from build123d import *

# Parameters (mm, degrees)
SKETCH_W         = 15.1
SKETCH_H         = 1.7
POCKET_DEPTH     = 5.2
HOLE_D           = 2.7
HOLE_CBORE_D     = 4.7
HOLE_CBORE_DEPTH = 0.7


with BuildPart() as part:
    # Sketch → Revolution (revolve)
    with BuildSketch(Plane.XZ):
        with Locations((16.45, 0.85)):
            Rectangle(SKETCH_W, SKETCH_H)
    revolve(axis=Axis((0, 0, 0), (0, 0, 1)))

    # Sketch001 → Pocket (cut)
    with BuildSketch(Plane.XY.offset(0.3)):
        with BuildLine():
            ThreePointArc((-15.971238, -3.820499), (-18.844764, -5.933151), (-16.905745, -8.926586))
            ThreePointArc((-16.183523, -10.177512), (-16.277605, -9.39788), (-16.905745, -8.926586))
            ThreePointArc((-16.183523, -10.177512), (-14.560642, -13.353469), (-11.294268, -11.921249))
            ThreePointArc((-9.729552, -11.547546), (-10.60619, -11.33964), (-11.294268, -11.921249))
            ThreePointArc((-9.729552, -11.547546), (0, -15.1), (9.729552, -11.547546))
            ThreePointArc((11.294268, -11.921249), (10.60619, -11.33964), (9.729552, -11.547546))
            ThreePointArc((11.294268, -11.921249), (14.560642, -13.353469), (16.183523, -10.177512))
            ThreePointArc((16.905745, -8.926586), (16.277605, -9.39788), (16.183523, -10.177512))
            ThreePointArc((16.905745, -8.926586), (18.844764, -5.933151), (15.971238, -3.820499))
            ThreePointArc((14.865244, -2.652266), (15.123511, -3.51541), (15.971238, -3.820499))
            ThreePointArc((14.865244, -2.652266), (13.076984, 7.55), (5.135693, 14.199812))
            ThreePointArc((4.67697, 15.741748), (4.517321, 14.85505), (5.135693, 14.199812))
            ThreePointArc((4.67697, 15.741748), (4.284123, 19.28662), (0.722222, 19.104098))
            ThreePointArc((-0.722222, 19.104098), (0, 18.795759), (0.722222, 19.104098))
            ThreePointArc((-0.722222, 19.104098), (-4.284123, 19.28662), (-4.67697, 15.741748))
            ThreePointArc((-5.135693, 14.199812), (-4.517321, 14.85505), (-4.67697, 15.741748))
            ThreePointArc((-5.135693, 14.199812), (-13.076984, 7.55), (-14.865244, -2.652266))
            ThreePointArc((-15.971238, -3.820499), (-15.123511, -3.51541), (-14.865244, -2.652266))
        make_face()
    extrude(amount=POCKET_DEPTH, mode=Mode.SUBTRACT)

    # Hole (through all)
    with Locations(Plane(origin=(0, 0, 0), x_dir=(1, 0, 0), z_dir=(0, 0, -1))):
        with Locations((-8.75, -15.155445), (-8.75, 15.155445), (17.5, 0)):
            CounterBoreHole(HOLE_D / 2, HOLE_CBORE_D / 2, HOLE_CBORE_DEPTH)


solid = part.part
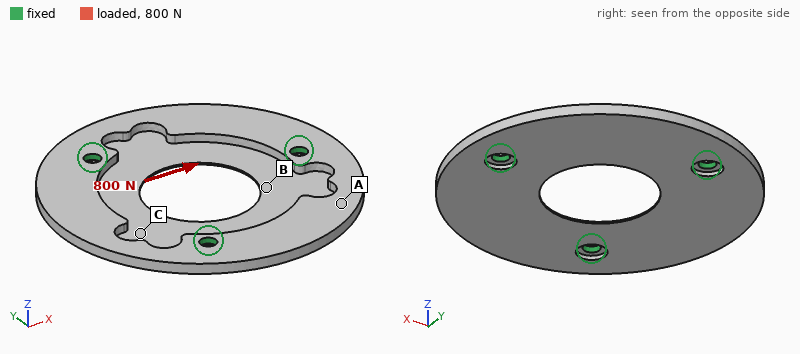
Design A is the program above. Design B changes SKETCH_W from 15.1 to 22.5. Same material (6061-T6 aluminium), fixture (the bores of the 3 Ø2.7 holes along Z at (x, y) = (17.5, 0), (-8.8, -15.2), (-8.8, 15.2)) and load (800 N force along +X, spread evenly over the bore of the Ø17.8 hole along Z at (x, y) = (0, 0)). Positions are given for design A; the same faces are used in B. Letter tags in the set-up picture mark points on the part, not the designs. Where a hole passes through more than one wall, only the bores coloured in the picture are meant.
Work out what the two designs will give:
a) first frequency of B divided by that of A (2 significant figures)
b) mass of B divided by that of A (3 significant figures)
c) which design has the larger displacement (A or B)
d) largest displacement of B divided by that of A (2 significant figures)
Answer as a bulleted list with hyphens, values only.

- 0.74
- 1.61
- B
- 1.2
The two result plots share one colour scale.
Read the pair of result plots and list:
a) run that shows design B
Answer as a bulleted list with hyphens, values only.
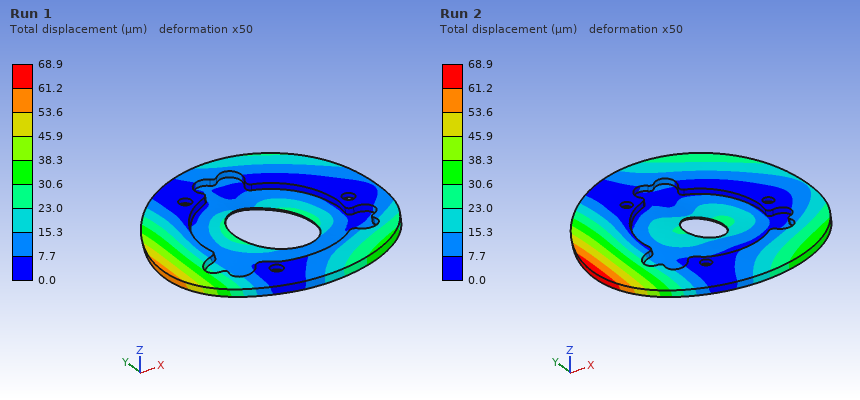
- Run 2
